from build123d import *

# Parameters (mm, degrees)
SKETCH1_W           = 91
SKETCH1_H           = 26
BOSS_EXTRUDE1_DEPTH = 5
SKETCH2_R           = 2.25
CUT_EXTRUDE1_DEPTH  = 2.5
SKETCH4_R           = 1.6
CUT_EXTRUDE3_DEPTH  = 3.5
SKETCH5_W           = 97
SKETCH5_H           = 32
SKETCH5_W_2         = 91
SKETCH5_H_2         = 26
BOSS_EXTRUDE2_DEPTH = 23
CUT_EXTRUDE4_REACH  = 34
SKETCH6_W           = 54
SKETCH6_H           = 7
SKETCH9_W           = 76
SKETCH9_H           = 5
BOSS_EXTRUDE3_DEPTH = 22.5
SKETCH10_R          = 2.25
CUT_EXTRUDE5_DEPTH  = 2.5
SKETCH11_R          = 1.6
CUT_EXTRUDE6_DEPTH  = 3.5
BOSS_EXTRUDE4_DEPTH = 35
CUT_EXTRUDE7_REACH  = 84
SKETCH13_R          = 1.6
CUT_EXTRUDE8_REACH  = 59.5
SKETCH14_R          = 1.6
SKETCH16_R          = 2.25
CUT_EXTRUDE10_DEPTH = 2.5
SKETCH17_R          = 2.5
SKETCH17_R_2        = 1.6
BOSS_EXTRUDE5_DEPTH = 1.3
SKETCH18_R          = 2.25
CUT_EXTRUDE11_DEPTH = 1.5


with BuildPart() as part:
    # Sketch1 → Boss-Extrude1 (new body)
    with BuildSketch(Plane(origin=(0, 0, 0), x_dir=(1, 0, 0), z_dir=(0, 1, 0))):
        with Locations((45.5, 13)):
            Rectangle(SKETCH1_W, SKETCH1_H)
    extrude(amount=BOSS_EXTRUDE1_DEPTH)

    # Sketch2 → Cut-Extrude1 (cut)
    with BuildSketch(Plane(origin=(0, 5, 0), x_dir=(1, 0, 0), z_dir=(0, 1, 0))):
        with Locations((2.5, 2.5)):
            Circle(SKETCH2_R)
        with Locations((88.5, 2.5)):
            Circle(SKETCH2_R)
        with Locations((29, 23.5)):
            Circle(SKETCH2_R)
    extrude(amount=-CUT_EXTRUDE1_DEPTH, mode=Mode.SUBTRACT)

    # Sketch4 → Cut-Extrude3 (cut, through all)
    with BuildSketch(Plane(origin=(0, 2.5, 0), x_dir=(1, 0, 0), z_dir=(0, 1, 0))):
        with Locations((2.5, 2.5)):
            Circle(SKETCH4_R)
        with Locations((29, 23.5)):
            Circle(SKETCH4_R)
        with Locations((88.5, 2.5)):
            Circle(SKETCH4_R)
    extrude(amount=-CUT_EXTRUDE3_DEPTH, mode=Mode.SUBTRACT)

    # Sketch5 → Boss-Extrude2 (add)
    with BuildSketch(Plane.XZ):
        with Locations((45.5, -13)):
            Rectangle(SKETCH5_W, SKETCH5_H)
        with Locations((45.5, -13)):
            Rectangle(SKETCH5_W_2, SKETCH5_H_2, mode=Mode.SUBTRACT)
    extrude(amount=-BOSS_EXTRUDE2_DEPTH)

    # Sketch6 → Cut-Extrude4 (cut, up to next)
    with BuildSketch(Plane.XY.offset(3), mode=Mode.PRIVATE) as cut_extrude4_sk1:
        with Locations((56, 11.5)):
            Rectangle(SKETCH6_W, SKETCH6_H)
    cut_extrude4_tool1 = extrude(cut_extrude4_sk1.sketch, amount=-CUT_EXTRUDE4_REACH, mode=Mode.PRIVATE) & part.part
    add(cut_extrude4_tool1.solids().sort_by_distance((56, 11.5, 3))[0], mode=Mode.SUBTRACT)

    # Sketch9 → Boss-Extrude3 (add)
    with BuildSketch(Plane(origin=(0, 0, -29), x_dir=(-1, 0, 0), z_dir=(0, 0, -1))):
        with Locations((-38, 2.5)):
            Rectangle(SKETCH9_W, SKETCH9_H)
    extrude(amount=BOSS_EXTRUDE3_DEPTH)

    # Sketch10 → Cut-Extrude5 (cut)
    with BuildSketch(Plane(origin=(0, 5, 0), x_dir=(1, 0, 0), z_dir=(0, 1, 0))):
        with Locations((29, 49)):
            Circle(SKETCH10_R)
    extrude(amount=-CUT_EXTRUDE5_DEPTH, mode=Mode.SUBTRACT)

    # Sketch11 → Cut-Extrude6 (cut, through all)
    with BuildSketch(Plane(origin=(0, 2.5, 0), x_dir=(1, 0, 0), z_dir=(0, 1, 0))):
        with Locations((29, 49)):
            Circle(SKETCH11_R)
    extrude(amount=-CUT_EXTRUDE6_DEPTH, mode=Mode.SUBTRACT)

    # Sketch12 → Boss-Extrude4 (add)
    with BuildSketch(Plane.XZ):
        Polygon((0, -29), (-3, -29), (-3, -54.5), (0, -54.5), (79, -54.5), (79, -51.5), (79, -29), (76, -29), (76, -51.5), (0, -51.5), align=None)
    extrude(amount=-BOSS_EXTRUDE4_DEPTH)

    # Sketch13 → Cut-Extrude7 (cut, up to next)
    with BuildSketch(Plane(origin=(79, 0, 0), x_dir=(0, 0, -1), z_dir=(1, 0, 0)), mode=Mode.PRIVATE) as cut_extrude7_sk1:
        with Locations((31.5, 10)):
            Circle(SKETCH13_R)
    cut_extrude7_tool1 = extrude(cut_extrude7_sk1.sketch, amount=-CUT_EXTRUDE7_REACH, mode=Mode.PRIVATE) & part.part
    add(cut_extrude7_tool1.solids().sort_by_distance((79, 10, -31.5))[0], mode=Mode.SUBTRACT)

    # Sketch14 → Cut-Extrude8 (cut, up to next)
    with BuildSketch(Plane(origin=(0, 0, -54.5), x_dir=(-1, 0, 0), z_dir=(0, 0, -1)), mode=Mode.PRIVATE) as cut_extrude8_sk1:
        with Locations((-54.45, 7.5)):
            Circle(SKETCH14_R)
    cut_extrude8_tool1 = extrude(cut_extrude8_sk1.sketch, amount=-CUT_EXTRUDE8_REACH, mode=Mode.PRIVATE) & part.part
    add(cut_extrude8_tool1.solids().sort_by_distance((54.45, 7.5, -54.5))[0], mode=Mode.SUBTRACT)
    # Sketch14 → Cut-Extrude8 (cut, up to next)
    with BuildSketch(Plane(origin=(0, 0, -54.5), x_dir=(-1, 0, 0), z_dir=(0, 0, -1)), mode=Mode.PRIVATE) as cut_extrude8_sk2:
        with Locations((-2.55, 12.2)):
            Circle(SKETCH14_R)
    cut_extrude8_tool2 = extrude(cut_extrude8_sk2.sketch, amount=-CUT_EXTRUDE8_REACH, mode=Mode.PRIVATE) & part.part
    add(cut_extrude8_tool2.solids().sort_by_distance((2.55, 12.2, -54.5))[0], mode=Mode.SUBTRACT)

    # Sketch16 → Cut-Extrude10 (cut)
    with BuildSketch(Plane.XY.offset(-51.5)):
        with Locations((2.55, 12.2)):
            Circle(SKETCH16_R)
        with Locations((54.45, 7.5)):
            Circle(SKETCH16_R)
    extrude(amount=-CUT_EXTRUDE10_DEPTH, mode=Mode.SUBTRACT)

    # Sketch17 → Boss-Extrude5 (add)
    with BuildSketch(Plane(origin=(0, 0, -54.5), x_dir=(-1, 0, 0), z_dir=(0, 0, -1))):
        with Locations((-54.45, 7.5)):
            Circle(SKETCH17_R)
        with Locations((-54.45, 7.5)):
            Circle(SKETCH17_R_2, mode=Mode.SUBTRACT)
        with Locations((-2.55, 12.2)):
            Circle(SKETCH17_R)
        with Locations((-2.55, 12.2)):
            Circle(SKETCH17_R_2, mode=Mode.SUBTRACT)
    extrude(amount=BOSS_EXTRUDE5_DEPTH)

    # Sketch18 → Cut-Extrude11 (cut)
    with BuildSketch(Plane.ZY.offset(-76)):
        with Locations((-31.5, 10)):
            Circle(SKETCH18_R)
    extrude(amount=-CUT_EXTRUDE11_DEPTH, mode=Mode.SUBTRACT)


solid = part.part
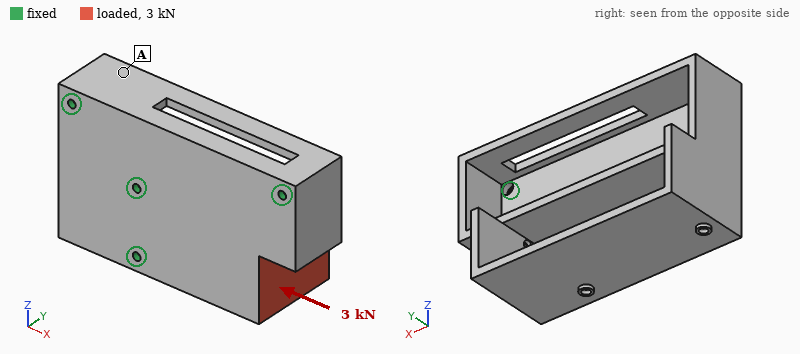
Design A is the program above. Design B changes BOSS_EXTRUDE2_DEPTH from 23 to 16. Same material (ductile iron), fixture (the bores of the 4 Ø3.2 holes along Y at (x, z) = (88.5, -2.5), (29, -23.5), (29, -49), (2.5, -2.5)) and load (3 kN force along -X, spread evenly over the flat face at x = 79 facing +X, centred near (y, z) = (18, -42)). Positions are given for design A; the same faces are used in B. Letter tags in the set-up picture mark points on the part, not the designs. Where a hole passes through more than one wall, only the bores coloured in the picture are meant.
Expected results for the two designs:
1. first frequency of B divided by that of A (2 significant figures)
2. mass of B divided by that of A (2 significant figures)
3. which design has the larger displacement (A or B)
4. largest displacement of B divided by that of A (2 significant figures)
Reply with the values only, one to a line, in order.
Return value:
0.98
0.90
B
1.6
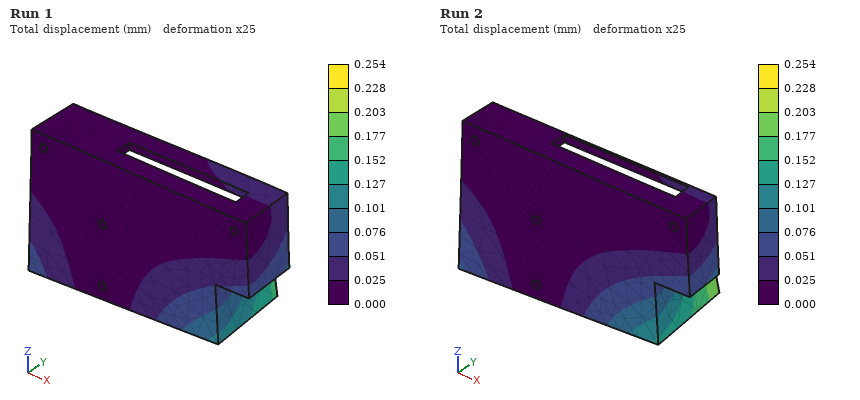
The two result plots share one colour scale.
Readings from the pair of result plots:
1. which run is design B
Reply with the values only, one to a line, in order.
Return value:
Run 2
